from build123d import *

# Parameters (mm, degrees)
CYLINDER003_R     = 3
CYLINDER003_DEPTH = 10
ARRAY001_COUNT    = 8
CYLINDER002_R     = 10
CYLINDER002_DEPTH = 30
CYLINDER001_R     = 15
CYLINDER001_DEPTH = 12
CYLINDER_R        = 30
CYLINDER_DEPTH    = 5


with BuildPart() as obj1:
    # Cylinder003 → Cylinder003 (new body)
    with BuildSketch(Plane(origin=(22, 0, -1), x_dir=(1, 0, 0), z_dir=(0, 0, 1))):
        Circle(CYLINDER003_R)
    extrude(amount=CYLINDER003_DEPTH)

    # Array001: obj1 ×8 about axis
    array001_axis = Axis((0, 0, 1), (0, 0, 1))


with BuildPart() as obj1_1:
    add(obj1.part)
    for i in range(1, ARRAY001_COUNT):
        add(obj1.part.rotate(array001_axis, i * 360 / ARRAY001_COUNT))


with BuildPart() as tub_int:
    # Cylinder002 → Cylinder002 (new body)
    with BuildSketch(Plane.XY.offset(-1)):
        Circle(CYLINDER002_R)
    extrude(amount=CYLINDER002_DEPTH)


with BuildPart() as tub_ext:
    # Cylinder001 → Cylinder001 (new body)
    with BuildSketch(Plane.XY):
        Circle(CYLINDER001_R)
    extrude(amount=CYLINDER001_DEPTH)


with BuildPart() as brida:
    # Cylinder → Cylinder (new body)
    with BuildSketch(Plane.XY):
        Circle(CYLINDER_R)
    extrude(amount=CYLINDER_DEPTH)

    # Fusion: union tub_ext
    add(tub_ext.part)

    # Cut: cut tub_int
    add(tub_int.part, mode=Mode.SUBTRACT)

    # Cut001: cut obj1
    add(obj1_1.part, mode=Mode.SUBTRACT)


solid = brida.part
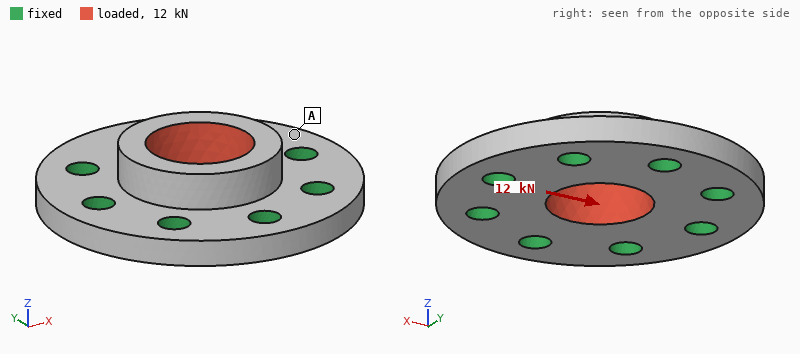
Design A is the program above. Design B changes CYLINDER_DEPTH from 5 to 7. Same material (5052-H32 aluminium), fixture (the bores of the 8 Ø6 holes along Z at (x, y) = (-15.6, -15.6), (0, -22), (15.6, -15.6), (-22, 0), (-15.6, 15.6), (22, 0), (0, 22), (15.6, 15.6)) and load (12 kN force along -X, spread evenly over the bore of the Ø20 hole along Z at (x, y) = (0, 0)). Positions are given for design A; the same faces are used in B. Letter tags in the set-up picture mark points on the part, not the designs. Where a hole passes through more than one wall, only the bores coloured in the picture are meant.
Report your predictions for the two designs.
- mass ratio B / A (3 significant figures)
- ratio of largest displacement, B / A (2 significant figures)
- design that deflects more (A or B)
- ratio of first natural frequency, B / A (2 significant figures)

1.27
0.65
A
1.2
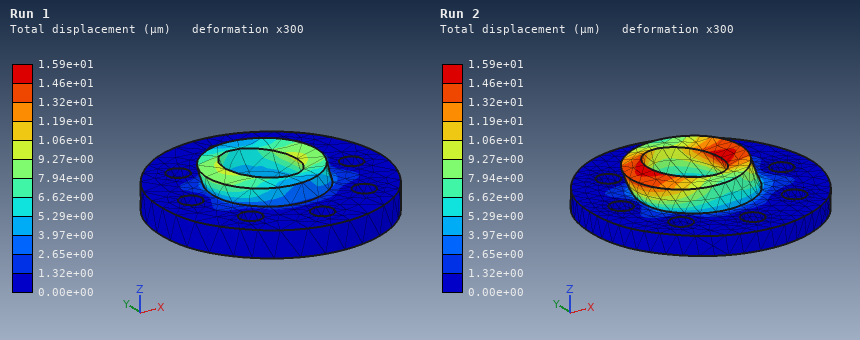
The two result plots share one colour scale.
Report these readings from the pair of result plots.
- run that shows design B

Run 1
